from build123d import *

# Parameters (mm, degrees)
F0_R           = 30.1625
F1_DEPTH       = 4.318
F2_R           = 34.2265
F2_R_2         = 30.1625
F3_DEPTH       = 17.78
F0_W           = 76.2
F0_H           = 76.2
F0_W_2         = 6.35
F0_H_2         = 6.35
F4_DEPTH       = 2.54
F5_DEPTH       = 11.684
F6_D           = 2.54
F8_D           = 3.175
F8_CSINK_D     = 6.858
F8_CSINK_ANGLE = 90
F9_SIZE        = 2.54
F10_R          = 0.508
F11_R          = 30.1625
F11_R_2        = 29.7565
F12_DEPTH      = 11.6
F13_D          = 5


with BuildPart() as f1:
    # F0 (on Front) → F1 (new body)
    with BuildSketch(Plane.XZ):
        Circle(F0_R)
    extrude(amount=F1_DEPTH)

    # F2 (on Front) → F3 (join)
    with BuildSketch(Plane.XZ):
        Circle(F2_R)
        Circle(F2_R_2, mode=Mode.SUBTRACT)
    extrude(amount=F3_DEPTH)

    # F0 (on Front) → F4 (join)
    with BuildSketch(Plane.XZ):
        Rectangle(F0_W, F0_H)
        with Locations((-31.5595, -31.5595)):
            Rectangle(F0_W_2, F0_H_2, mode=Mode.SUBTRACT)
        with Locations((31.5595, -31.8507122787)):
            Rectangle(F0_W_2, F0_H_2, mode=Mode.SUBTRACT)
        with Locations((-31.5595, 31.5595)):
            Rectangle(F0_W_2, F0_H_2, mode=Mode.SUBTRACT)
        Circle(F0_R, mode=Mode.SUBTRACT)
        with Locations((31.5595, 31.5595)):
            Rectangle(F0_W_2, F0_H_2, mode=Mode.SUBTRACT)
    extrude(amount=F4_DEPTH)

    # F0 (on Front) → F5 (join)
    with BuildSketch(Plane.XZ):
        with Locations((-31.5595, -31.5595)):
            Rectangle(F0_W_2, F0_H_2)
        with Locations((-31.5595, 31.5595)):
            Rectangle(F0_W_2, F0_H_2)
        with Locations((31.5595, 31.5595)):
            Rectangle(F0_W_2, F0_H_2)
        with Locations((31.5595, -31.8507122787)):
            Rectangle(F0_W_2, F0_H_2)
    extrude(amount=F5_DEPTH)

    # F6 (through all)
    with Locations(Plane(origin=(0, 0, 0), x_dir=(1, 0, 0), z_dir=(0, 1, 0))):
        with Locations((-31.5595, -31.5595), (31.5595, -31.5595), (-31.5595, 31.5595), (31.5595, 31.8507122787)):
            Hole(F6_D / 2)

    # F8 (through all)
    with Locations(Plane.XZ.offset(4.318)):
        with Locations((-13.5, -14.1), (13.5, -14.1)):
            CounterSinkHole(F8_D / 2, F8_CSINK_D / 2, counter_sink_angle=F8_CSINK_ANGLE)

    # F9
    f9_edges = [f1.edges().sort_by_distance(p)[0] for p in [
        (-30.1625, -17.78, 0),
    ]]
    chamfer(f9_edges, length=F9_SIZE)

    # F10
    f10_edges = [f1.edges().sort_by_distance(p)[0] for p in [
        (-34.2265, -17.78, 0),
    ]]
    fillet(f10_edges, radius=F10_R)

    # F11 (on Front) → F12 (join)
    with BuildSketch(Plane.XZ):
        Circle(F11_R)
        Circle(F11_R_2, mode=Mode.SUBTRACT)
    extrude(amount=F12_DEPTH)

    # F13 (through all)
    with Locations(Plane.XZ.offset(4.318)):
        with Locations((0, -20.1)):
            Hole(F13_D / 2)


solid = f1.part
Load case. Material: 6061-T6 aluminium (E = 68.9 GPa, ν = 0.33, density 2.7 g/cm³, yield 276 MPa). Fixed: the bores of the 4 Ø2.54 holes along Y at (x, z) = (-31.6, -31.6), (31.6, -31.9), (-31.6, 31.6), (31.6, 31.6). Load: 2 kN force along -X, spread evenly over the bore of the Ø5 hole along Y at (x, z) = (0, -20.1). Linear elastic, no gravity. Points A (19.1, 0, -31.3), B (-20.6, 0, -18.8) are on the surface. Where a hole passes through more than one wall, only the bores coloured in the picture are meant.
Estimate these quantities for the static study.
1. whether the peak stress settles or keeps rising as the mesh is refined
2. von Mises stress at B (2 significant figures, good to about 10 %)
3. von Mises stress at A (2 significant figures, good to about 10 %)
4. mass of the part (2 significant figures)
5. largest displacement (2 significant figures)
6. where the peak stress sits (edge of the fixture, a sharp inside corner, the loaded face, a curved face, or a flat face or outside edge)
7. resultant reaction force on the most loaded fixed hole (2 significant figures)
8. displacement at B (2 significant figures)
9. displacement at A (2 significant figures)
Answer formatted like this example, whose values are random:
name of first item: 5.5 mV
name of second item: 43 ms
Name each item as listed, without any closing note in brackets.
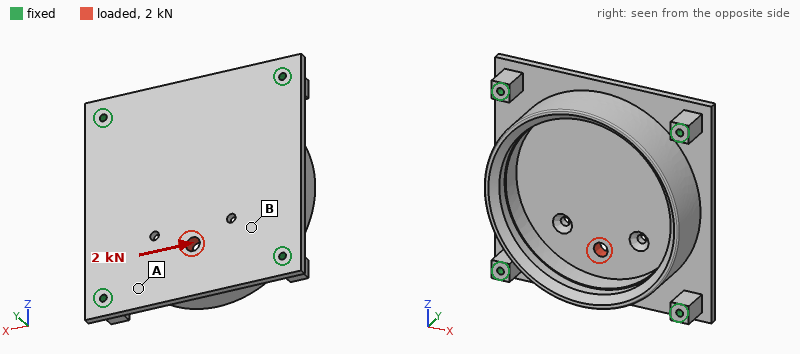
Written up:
whether the peak stress settles or keeps rising as the mesh is refined: keeps rising
von Mises stress at B: 6.8 MPa
von Mises stress at A: 15 MPa
mass of the part: 90 g
largest displacement: 9.0 µm
where the peak stress sits: edge of the fixture
resultant reaction force on the most loaded fixed hole: 750 N
displacement at B: 5.2 µm
displacement at A: 4.0 µm
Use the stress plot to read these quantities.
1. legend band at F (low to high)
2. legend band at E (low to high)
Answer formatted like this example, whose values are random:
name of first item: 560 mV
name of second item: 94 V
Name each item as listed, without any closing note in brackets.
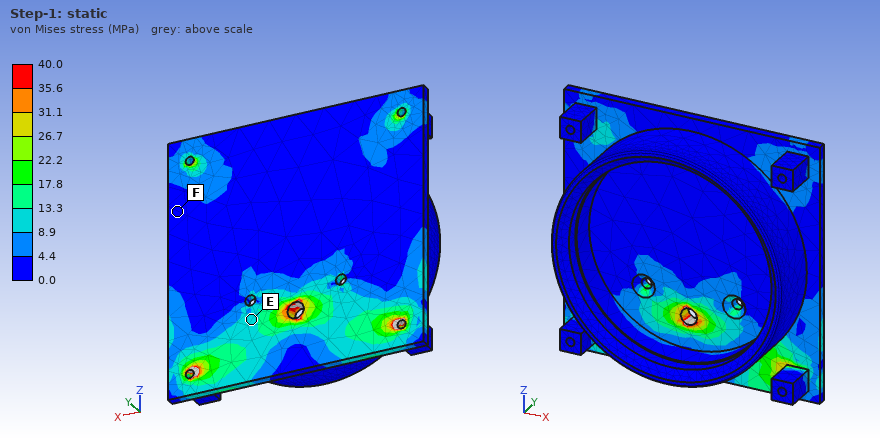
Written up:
legend band at F: 0.0 to 4.4 MPa
legend band at E: 8.9 to 13.3 MPa
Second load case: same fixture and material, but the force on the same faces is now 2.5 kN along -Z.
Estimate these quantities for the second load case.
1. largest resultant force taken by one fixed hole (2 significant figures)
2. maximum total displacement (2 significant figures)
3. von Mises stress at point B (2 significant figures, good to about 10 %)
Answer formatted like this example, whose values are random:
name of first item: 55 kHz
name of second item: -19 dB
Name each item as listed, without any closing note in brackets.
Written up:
largest resultant force taken by one fixed hole: 700 N
maximum total displacement: 15 µm
von Mises stress at point B: 8.3 MPa
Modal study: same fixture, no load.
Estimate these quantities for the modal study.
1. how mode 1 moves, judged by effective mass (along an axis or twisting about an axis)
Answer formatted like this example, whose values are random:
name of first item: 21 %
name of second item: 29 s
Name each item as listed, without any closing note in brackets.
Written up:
how mode 1 moves, judged by effective mass: along Y
